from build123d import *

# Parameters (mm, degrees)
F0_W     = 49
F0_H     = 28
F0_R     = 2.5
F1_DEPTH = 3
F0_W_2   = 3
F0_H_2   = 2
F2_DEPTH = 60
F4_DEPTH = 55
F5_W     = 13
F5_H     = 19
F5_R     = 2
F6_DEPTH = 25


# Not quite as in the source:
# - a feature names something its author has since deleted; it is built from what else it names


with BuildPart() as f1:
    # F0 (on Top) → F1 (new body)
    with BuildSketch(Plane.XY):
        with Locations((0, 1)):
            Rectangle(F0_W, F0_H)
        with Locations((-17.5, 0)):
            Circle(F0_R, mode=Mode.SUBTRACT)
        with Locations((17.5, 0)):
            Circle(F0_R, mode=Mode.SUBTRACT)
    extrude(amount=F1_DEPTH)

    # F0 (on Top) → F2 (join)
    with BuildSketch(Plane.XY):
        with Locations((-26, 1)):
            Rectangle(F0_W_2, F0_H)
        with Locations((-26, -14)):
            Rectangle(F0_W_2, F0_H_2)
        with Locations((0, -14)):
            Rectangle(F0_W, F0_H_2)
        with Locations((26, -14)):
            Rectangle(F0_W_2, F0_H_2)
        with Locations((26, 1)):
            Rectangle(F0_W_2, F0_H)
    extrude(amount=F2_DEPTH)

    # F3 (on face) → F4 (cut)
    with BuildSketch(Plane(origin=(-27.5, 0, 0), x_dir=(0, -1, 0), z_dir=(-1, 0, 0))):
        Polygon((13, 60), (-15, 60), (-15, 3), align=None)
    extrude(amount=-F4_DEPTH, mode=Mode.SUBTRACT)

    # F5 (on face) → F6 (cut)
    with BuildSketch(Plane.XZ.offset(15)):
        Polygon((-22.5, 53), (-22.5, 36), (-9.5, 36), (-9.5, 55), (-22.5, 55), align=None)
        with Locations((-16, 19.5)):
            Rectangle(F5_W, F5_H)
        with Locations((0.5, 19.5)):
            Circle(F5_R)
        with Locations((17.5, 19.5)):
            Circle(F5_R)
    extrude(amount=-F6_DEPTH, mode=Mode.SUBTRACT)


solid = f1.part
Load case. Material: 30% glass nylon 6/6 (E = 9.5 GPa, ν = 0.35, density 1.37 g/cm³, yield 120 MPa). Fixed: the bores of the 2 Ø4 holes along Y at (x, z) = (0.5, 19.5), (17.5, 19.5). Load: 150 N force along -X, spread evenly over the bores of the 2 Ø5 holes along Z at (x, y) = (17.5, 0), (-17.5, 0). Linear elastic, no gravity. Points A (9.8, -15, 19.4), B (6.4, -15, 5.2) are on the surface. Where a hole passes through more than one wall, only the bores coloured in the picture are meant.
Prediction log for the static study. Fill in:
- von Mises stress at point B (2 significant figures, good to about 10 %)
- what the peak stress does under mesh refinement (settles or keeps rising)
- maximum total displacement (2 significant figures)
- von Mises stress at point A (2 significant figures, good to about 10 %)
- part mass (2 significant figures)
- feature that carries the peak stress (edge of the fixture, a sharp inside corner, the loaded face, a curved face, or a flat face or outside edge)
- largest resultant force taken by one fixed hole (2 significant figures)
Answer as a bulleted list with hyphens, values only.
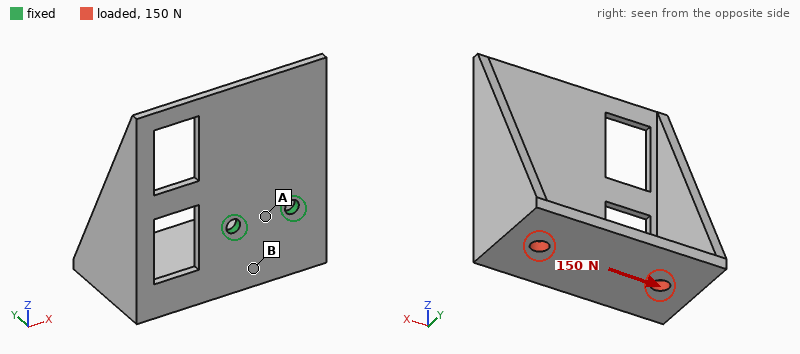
- 11 MPa
- keeps rising
- 0.79 mm
- 5.6 MPa
- 20 g
- edge of the fixture
- 180 N
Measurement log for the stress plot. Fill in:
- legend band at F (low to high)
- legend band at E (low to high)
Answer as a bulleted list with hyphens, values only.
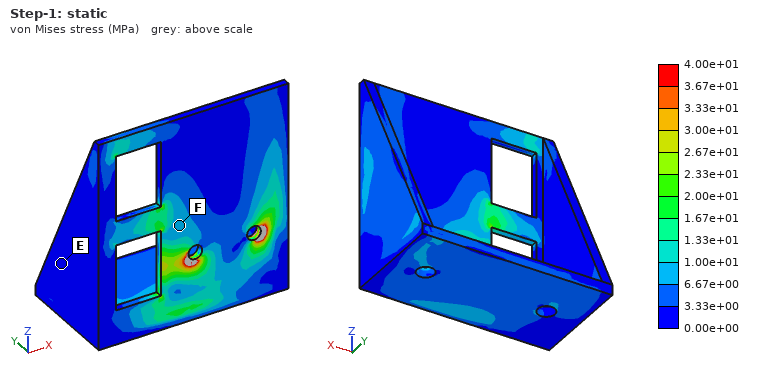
- 6.67e+00 to 1.00e+01 MPa
- 0.00e+00 to 3.33e+00 MPa
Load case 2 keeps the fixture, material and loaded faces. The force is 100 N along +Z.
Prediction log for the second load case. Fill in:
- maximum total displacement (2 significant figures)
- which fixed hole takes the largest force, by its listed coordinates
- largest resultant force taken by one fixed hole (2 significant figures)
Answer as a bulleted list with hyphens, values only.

- 0.99 mm
- (0.5, 19.5)
- 98 N
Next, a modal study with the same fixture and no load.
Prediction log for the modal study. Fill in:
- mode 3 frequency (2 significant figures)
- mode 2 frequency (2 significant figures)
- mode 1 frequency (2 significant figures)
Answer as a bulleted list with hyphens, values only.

- 990 Hz
- 560 Hz
- 470 Hz
